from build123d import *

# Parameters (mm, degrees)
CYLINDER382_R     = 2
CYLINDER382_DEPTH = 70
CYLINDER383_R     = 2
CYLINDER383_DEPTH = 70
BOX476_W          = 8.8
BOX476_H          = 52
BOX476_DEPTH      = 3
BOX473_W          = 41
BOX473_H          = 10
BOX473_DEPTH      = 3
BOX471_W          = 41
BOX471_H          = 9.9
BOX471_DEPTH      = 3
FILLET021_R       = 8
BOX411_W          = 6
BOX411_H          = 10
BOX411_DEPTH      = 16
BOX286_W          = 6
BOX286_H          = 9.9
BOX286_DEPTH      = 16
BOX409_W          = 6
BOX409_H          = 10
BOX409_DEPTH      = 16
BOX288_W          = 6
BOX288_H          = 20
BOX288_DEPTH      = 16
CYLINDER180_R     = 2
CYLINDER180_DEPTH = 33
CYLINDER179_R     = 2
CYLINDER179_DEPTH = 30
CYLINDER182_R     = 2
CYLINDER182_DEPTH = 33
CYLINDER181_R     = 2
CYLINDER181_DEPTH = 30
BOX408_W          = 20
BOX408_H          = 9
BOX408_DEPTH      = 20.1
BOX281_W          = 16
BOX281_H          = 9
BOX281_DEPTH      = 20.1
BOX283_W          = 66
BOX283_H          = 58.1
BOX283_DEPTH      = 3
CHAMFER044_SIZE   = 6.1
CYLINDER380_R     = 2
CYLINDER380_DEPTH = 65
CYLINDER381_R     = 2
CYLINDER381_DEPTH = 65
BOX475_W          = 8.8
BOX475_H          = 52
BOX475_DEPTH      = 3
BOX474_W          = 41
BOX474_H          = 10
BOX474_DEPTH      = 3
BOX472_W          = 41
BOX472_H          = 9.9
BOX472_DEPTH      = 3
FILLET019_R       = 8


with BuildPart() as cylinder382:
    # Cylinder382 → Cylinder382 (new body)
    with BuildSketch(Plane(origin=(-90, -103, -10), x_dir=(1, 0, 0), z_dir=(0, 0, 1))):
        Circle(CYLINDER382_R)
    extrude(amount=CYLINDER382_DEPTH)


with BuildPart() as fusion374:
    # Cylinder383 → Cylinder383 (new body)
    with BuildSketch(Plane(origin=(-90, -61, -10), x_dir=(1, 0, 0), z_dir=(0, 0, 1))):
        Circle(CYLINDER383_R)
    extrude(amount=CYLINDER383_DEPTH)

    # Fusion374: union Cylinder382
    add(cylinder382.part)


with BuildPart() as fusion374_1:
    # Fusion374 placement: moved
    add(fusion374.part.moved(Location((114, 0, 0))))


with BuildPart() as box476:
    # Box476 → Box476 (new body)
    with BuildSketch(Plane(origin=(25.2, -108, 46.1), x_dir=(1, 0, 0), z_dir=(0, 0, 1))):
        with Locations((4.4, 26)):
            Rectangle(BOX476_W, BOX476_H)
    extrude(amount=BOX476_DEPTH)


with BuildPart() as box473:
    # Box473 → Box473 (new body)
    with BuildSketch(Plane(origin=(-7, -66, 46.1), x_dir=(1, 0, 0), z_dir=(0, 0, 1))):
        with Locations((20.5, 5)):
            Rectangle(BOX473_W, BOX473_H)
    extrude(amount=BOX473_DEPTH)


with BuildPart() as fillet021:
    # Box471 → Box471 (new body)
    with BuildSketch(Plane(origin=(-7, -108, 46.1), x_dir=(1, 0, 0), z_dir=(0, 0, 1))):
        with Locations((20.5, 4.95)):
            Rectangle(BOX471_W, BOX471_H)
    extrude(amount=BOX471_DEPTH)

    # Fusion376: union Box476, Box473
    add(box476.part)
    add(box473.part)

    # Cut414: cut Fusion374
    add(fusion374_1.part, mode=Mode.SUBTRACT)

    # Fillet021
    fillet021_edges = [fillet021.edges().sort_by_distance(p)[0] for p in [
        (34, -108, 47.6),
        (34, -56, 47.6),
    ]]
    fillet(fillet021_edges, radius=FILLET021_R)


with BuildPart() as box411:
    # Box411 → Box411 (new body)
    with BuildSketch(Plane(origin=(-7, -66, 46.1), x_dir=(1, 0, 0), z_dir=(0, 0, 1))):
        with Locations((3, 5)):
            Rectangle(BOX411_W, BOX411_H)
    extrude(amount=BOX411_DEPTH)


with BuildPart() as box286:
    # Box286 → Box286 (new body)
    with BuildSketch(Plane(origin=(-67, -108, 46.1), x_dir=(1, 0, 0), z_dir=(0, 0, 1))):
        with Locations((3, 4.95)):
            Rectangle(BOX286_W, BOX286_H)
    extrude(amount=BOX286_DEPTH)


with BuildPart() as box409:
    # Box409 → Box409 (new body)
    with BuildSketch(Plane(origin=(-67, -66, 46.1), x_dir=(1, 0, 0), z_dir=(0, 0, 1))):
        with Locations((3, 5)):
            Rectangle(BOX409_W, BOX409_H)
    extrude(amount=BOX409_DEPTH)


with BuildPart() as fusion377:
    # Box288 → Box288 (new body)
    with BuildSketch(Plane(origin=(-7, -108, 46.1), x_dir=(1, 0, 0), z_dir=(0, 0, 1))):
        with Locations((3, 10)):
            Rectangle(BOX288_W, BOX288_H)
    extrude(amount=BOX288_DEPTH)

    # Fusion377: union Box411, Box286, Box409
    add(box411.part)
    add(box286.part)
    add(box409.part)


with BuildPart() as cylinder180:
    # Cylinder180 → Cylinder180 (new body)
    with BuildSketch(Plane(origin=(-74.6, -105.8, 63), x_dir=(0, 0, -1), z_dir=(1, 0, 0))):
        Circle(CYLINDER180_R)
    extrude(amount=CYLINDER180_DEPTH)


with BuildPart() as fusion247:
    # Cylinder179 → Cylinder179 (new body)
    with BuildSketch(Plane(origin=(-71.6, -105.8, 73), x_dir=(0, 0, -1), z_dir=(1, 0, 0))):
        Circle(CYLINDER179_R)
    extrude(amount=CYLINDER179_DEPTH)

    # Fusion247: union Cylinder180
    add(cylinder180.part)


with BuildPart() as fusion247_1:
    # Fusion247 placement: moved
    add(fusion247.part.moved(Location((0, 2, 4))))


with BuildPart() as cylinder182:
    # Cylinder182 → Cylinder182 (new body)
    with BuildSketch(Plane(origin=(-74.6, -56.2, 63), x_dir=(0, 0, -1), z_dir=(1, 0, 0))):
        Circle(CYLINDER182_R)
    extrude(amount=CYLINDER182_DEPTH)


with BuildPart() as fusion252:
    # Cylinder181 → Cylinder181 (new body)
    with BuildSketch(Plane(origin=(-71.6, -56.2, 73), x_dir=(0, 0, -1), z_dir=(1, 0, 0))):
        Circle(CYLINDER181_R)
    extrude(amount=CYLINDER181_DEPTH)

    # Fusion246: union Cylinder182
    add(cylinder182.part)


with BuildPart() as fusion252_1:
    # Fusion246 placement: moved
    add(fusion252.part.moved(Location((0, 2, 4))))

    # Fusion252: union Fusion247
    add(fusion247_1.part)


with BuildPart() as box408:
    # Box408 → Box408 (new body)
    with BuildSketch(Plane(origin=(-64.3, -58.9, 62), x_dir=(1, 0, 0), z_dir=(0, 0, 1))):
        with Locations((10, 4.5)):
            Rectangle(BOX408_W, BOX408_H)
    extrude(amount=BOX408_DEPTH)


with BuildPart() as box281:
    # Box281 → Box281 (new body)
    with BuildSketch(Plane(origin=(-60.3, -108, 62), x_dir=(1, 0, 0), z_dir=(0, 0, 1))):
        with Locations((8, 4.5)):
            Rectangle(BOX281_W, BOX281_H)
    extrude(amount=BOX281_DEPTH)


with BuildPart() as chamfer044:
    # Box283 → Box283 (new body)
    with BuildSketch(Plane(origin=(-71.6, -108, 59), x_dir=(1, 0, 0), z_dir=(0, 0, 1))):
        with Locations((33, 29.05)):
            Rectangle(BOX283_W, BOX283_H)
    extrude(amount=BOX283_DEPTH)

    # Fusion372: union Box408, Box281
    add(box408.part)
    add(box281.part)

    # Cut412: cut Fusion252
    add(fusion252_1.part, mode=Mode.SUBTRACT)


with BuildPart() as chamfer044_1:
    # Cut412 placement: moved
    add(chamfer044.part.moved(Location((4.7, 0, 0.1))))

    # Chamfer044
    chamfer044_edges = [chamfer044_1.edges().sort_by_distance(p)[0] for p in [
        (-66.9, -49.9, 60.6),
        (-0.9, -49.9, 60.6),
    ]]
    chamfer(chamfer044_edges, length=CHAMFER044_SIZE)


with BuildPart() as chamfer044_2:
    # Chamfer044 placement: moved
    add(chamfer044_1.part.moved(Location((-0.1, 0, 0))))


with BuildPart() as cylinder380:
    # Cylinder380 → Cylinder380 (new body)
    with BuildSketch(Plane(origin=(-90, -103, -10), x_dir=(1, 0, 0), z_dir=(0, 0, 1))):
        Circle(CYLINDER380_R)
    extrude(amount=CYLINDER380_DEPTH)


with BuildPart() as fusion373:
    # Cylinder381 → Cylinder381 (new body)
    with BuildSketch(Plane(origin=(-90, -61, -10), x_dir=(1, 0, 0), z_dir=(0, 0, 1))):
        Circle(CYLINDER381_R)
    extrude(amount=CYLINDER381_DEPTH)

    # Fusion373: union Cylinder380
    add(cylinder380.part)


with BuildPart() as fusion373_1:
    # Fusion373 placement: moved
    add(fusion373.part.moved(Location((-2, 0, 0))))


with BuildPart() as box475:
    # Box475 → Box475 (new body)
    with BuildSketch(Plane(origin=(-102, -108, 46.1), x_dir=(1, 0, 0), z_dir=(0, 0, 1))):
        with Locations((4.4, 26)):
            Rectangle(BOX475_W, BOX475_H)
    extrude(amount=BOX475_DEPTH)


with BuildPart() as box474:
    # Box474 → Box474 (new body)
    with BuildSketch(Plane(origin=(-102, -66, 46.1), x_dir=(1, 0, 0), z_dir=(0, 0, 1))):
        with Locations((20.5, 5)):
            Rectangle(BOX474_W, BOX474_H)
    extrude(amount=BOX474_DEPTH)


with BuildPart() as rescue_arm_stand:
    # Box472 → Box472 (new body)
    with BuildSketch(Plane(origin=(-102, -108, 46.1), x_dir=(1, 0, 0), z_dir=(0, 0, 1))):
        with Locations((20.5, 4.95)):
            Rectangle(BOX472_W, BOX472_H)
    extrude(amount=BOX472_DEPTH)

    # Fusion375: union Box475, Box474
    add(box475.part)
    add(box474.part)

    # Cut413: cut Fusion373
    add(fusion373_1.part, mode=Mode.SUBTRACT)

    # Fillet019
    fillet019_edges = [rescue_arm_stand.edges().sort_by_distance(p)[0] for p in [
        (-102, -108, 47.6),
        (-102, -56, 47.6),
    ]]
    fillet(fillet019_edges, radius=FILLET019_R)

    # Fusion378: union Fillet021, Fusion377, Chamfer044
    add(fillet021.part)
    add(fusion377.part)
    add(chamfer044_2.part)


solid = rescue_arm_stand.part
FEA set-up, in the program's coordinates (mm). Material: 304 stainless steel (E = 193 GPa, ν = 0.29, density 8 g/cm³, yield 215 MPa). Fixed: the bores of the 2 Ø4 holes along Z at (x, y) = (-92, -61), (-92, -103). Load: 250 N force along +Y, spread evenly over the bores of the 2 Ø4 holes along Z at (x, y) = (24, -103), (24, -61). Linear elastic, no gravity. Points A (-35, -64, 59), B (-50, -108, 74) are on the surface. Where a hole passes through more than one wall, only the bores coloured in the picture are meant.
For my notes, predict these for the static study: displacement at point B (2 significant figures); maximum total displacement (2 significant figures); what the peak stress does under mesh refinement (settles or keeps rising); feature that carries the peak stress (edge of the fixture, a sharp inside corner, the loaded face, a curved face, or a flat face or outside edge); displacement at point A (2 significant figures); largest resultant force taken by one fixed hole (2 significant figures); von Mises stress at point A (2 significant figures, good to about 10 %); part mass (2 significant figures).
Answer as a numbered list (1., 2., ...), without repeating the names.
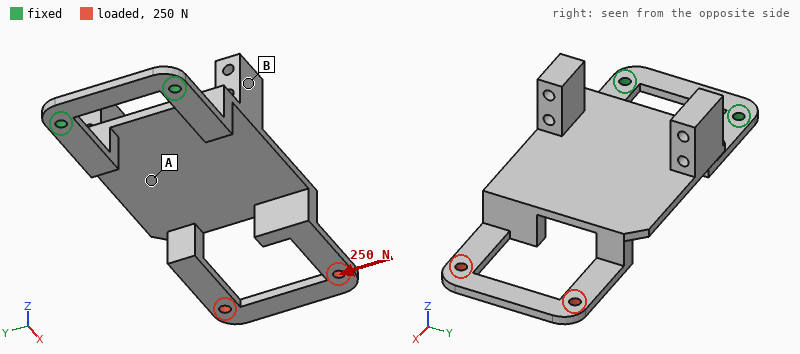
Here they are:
1. 0.18 mm
2. 0.57 mm
3. keeps rising
4. edge of the fixture
5. 0.19 mm
6. 490 N
7. 42 MPa
8. 210 g
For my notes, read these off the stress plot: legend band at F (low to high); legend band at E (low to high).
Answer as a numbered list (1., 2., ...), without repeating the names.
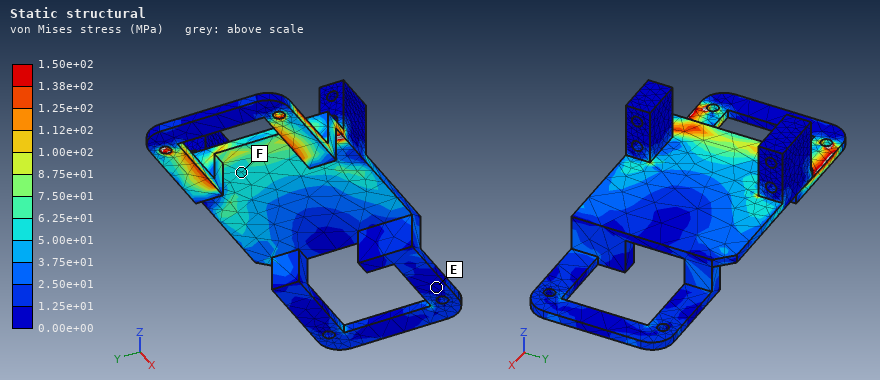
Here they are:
1. 5.00e+01 to 6.25e+01 MPa
2. 0.00e+00 to 1.25e+01 MPa
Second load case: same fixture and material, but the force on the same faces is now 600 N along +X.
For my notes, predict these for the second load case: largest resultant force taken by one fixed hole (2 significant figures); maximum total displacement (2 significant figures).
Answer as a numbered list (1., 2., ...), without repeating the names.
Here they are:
1. 320 N
2. 1.1 mm
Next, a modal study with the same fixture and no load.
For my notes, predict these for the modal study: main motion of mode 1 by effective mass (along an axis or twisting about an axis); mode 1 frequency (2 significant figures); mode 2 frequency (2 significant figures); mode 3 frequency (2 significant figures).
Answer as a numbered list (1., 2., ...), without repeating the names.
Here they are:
1. along Z
2. 110 Hz
3. 470 Hz
4. 670 Hz
